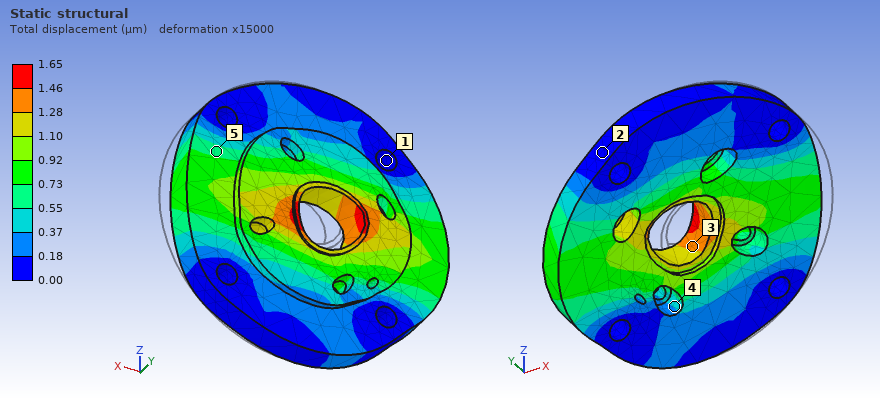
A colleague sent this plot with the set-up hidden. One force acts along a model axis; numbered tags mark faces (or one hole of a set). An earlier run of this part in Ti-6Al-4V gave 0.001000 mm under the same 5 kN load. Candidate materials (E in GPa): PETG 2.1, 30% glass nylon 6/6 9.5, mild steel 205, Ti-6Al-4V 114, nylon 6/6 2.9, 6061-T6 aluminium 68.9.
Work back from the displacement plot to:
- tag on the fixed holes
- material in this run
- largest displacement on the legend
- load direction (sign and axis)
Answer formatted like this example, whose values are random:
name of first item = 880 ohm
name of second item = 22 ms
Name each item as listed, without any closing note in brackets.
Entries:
tag on the fixed holes = 1
material in this run = 6061-T6 aluminium
largest displacement on the legend = 1.65 µm
load direction = -X
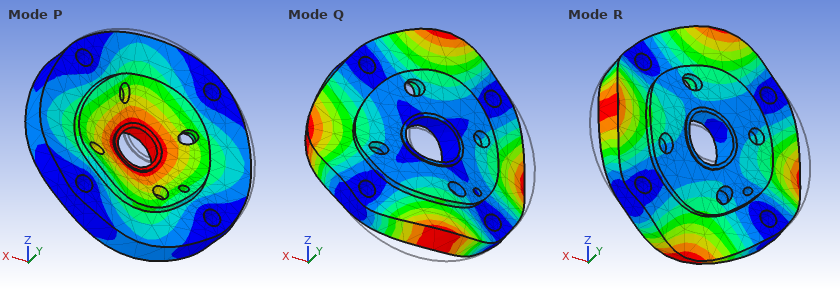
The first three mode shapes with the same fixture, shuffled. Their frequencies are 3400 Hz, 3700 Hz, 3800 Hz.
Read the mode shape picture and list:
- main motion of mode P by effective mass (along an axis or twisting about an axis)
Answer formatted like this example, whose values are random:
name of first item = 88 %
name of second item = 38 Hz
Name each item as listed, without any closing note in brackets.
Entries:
main motion of mode P by effective mass = along Y
